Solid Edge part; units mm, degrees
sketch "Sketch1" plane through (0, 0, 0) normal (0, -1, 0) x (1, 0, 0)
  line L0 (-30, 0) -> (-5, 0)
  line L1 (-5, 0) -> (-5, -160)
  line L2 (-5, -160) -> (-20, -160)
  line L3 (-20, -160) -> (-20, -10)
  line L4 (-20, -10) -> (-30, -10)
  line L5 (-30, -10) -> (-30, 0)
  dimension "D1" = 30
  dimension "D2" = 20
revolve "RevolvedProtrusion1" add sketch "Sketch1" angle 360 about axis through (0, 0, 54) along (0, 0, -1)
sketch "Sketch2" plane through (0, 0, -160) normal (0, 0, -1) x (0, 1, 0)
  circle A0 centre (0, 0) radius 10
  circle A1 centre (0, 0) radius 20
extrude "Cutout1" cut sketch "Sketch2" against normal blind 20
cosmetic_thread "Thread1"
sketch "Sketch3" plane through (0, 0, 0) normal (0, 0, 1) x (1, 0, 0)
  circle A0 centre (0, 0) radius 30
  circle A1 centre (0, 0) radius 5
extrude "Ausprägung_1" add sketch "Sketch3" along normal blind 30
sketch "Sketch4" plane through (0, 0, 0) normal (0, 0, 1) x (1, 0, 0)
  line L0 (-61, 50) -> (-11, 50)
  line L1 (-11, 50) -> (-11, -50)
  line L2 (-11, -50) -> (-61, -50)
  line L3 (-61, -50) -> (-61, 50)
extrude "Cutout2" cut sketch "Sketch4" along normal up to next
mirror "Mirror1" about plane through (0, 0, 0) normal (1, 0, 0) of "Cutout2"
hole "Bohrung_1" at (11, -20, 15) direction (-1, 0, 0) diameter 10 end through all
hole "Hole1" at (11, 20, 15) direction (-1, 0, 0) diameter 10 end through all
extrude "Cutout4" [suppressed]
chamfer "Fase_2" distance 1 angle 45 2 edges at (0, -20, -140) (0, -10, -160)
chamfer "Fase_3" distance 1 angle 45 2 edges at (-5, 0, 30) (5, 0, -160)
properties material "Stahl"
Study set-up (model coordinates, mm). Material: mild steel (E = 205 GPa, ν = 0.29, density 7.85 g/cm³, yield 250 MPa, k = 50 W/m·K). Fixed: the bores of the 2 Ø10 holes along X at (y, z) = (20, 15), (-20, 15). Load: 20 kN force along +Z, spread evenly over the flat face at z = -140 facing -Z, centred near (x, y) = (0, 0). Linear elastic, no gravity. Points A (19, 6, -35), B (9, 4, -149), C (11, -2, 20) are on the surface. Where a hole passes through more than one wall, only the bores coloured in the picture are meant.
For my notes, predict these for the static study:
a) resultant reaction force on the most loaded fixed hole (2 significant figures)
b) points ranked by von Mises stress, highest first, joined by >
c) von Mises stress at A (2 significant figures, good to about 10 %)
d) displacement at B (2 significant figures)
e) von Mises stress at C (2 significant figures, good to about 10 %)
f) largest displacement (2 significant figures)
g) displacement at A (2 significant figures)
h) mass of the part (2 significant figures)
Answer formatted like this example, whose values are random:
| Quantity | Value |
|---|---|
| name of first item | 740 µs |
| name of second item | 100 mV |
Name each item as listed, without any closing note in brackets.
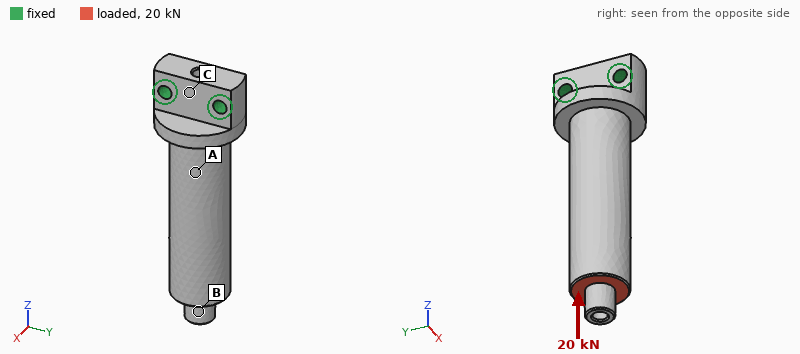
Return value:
| Quantity | Value |
|---|---|
| resultant reaction force on the most loaded fixed hole | 10 kN |
| points ranked by von Mises stress, highest first, joined by > | A > C > B |
| von Mises stress at A | 17 MPa |
| displacement at B | 13 µm |
| von Mises stress at C | 5.5 MPa |
| largest displacement | 14 µm |
| displacement at A | 4.7 µm |
| mass of the part | 1.7 kg |
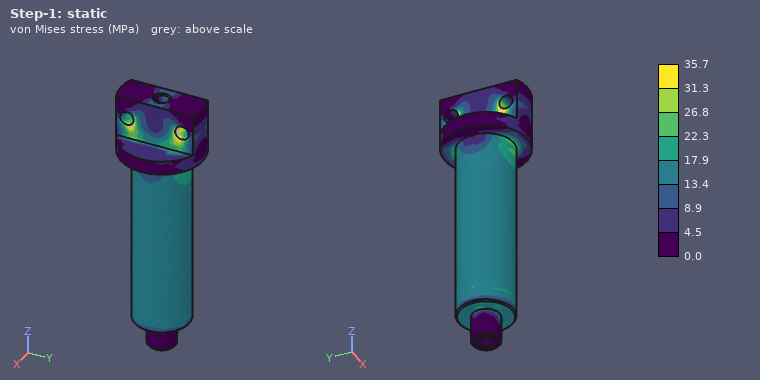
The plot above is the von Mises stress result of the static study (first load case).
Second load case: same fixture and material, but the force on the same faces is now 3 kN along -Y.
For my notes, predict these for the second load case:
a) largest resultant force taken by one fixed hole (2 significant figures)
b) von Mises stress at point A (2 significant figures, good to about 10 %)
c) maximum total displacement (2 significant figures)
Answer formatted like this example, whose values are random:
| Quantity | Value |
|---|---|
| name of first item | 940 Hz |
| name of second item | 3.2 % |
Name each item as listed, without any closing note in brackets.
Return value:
| Quantity | Value |
|---|---|
| largest resultant force taken by one fixed hole | 11 kN |
| von Mises stress at point A | 16 MPa |
| maximum total displacement | 0.14 mm |
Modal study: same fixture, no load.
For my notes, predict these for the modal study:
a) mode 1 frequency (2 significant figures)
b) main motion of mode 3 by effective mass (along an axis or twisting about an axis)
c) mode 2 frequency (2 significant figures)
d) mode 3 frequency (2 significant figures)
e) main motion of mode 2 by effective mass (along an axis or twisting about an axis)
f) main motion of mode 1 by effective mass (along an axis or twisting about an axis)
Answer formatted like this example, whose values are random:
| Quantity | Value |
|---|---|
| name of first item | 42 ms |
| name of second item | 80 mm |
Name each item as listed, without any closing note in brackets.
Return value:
| Quantity | Value |
|---|---|
| mode 1 frequency | 860 Hz |
| main motion of mode 3 by effective mass | twisting about Z |
| mode 2 frequency | 1300 Hz |
| mode 3 frequency | 5300 Hz |
| main motion of mode 2 by effective mass | along Y |
| main motion of mode 1 by effective mass | along X |
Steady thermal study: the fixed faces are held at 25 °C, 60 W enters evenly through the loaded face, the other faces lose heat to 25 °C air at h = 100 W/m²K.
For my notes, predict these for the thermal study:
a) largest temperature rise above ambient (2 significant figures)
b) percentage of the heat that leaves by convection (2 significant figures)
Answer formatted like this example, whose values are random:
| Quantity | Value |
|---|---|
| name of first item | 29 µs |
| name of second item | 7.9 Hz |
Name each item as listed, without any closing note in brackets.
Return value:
| Quantity | Value |
|---|---|
| largest temperature rise above ambient | 54 K |
| percentage of the heat that leaves by convection | 87 % |
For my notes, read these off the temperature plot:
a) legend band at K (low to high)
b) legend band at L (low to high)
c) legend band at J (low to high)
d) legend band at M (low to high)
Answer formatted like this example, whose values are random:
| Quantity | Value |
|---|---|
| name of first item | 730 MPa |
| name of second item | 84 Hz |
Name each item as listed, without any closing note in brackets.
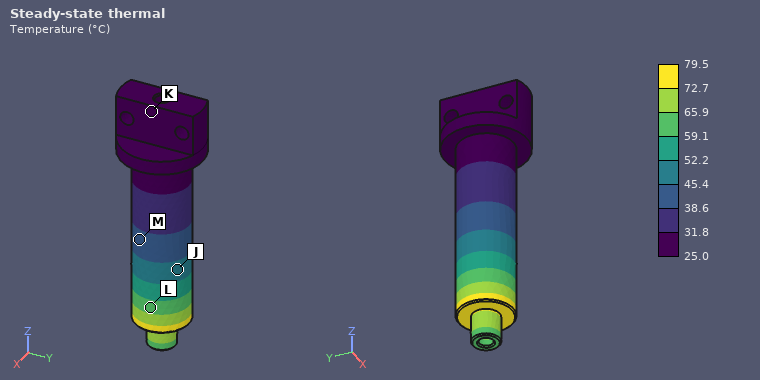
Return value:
| Quantity | Value |
|---|---|
| legend band at K | 25.0 to 31.8 °C |
| legend band at L | 59.1 to 65.9 °C |
| legend band at J | 45.4 to 52.2 °C |
| legend band at M | 38.6 to 45.4 °C |
